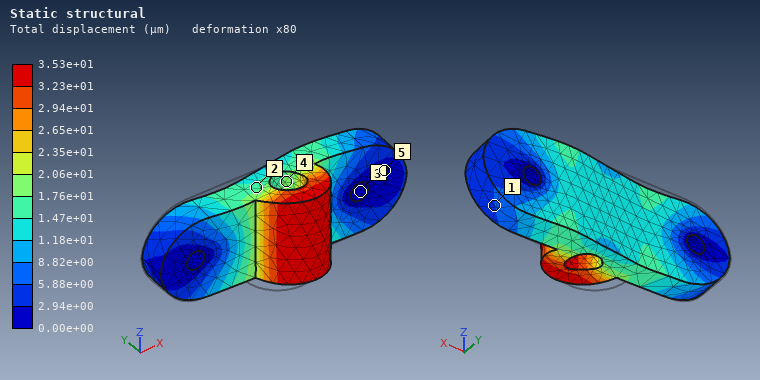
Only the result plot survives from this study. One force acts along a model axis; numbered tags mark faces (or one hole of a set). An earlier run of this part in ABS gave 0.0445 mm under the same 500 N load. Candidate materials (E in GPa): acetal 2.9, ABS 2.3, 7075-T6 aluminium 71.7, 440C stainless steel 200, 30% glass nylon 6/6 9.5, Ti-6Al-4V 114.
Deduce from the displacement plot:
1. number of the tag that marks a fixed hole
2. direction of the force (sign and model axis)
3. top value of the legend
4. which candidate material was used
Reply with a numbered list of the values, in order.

1. 3
2. +X
3. 3.53e+01 µm
4. acetal
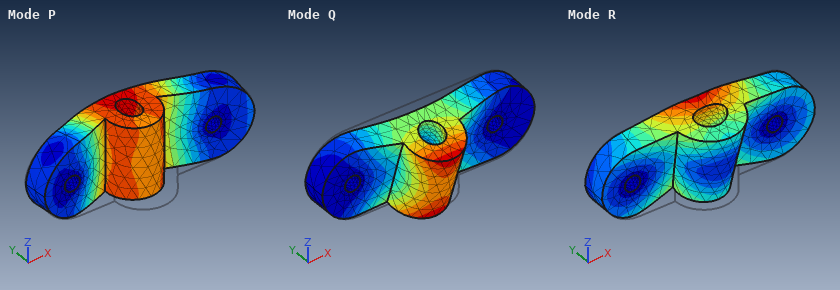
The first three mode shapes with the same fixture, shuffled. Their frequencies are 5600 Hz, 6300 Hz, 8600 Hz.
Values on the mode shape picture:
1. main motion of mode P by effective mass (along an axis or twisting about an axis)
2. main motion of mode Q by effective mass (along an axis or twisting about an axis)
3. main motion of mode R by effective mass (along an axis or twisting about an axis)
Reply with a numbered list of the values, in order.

1. along Y
2. along Z
3. along Z
